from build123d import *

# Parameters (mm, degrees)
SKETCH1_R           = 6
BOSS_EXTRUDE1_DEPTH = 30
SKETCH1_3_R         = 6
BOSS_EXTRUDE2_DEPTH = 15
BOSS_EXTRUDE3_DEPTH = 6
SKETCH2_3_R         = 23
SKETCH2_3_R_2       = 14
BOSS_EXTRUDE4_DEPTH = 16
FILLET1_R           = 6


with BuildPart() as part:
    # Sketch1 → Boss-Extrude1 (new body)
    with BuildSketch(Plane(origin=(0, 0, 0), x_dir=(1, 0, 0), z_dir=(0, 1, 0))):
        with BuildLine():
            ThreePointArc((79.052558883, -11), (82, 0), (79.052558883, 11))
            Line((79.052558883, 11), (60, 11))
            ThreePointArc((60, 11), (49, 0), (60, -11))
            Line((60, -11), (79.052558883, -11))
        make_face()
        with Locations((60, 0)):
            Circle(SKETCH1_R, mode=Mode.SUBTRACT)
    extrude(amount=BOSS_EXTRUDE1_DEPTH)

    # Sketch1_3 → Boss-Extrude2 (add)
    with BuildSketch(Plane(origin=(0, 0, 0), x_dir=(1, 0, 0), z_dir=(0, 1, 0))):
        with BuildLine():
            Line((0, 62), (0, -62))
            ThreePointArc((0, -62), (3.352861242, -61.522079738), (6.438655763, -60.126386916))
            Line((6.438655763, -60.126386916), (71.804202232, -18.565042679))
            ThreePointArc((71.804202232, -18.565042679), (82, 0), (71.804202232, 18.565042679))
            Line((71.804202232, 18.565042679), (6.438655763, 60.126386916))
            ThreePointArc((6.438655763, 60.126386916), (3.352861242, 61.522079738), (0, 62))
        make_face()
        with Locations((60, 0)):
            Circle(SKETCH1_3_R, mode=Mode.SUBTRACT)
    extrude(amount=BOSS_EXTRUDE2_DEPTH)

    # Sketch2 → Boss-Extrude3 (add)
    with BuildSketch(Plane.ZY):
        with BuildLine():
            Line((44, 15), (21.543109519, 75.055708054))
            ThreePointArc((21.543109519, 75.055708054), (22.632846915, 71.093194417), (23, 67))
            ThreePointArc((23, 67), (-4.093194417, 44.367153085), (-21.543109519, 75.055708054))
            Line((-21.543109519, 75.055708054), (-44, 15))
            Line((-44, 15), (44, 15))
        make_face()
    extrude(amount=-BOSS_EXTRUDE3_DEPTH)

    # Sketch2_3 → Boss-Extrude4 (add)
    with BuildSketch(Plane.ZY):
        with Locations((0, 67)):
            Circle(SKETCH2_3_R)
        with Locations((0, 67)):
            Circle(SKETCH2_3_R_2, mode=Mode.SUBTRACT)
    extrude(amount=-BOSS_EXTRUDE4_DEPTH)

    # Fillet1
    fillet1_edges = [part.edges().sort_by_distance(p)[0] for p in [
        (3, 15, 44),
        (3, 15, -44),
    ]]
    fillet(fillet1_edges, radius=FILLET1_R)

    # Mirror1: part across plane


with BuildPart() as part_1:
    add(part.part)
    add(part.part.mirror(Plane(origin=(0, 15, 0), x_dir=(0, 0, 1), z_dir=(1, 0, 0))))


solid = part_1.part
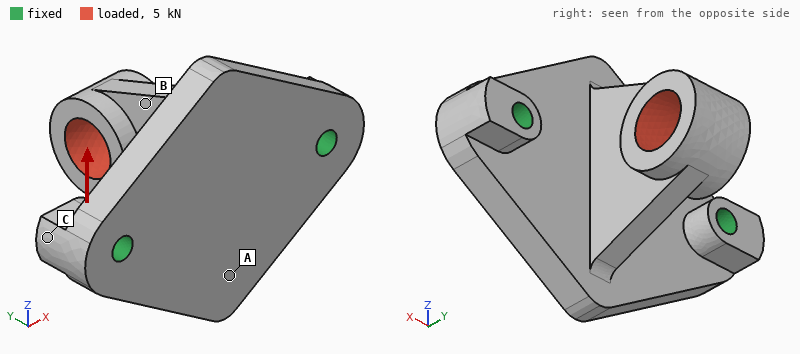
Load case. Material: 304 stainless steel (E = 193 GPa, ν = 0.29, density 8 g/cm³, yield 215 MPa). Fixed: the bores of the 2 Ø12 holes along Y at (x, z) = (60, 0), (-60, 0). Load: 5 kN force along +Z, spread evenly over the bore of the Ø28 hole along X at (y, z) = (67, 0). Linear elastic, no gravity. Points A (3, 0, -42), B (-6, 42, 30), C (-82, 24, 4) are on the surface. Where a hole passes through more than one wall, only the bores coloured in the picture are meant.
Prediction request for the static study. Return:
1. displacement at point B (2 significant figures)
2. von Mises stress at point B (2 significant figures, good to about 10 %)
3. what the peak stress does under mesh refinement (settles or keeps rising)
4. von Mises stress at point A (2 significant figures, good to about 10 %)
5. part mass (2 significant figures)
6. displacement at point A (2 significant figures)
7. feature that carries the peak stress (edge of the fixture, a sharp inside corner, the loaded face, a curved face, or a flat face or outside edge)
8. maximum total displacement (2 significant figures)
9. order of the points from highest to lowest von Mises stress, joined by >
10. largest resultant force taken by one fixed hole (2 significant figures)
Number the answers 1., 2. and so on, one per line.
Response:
1. 0.053 mm
2. 16 MPa
3. keeps rising
4. 29 MPa
5. 2.1 kg
6. 0.044 mm
7. edge of the fixture
8. 0.10 mm
9. A > B > C
10. 2.5 kN
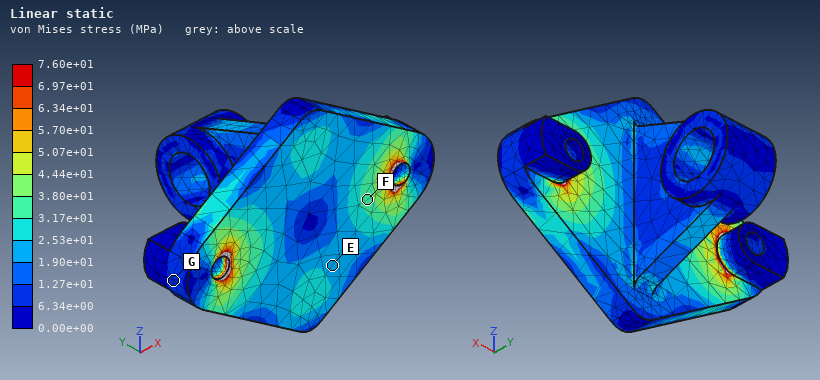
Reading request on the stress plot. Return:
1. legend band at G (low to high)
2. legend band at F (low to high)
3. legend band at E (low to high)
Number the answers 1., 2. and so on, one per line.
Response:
1. 6.34e+00 to 1.27e+01 MPa
2. 3.17e+01 to 3.80e+01 MPa
3. 1.90e+01 to 2.53e+01 MPa
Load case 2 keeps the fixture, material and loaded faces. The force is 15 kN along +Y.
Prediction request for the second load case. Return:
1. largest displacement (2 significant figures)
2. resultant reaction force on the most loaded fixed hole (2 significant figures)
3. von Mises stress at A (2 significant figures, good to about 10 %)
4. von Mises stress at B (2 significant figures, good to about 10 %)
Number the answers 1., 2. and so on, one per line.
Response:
1. 44 µm
2. 7.5 kN
3. 35 MPa
4. 16 MPa
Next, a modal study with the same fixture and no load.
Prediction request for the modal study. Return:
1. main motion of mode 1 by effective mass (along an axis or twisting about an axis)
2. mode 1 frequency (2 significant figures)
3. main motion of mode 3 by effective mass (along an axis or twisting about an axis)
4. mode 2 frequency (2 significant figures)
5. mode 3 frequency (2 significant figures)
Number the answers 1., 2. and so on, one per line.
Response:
1. along X
2. 1500 Hz
3. along Y
4. 1700 Hz
5. 2900 Hz
